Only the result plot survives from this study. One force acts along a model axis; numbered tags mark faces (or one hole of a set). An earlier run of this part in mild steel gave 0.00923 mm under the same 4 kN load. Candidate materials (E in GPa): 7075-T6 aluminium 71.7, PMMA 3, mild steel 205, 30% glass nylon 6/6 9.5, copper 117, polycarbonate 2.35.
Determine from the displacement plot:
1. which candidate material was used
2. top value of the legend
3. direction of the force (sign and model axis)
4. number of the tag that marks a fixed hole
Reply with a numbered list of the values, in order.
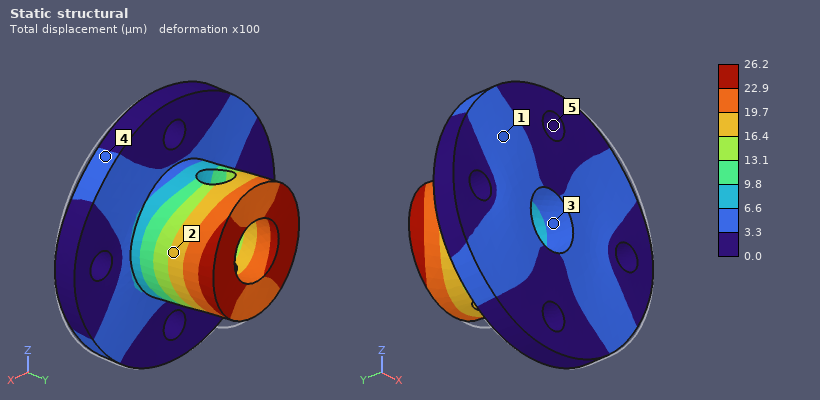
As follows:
1. 7075-T6 aluminium
2. 26.2 µm
3. -X
4. 5
